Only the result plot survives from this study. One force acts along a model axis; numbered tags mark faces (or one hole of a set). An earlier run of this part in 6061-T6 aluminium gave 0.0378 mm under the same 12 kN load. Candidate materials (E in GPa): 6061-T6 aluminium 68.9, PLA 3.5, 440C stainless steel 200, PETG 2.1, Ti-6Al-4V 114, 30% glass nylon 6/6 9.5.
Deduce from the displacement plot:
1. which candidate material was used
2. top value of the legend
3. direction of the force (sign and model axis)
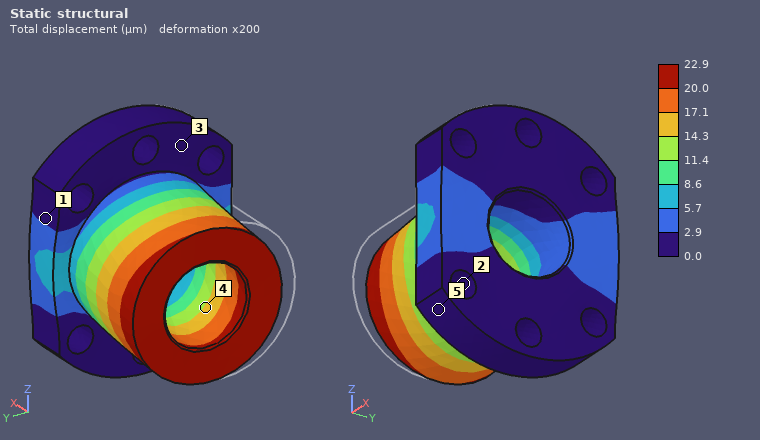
Ti-6Al-4V
22.9 µm
+Y
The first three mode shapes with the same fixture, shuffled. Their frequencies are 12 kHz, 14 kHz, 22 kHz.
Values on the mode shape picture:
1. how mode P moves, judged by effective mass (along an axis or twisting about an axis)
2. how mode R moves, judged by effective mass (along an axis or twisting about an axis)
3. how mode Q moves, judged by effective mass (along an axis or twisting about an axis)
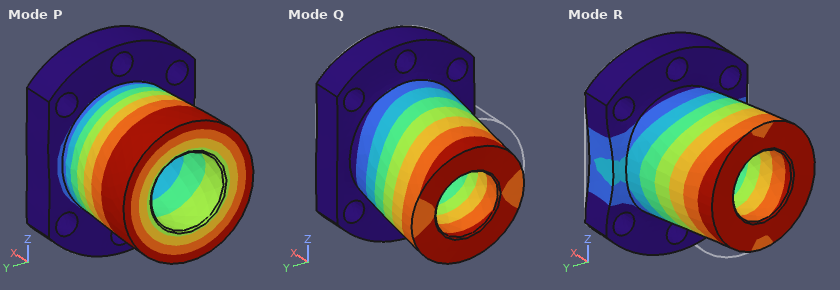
twisting about X
along Y
along Z
